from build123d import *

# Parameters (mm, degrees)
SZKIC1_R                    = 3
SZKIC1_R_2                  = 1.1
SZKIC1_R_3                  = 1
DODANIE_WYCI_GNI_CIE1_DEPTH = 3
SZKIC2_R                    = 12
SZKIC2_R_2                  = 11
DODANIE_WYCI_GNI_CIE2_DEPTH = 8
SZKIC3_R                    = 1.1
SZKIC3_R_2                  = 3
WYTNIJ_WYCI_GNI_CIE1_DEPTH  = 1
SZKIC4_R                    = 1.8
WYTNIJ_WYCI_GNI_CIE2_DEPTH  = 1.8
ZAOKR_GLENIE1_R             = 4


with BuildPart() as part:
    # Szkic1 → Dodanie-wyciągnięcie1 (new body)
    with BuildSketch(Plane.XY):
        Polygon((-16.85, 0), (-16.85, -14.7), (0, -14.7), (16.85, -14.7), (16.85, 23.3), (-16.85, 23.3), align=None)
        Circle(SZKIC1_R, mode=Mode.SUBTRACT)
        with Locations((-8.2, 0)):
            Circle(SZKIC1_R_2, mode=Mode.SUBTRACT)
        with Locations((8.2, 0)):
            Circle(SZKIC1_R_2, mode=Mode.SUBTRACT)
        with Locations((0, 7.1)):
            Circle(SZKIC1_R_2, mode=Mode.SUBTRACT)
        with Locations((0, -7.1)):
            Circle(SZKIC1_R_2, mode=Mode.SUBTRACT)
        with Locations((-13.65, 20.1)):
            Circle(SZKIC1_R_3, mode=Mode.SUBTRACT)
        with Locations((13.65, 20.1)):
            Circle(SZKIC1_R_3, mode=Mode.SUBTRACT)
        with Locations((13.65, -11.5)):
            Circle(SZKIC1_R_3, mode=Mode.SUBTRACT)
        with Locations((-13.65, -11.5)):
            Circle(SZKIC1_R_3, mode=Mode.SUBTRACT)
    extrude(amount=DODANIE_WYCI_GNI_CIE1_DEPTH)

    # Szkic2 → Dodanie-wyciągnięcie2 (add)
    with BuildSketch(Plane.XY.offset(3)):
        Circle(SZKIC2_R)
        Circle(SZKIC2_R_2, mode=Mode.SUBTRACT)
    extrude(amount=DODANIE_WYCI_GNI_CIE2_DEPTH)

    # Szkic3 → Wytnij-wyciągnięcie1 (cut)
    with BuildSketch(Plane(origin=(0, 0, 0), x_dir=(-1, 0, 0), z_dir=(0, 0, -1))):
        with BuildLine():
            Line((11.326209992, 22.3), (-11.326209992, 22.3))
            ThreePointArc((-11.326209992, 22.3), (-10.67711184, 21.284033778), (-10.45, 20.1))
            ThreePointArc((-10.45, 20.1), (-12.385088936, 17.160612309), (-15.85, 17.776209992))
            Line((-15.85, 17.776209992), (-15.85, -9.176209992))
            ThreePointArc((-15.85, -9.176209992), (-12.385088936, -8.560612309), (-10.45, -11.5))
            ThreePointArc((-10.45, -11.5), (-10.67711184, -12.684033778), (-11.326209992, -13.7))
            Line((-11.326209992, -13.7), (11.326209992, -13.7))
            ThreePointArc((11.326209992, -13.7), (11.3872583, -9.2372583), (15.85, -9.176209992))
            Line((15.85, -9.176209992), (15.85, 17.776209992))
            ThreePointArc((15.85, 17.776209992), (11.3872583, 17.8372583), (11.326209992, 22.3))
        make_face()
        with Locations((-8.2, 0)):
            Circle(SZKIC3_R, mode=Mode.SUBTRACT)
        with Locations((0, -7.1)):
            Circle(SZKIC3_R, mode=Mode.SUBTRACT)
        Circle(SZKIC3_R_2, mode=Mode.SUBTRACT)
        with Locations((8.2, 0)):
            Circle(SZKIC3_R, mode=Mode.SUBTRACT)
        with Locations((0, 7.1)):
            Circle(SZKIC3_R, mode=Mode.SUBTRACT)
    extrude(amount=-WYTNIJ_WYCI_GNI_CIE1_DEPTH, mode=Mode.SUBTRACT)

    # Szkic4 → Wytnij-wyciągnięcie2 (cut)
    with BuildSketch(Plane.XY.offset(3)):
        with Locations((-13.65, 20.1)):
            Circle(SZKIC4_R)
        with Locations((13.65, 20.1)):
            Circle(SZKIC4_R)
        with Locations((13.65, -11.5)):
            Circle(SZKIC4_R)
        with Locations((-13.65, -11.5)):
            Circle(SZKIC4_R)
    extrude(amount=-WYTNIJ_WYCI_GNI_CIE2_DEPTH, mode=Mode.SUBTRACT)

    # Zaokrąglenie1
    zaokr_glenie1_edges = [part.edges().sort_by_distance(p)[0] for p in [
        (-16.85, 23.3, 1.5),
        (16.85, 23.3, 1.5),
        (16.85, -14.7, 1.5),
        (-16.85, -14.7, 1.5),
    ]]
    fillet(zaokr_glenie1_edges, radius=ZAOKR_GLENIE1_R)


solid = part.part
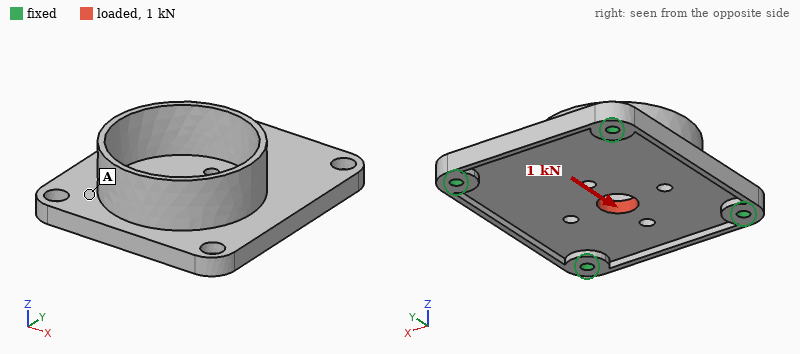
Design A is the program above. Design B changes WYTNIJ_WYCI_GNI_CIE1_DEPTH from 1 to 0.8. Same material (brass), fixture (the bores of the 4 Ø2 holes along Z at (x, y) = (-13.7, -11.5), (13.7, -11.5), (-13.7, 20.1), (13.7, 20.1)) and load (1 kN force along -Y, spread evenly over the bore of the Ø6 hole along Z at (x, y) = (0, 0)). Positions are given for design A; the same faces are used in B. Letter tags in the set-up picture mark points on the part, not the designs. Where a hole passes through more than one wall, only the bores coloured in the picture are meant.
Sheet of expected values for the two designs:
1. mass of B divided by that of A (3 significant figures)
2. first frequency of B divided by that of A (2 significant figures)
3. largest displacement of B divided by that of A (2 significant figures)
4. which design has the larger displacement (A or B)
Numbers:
1.06
1.0
0.90
A
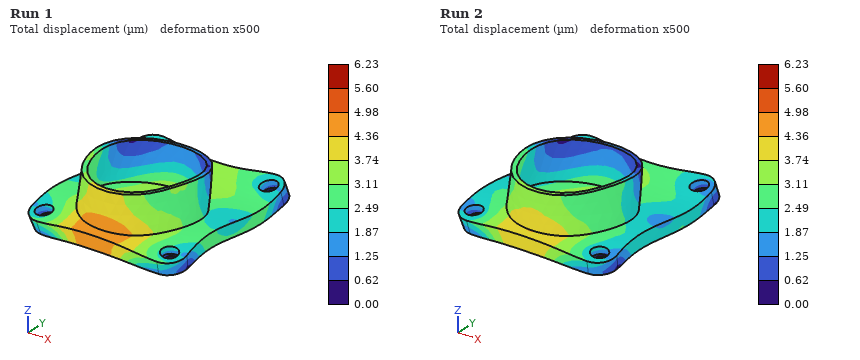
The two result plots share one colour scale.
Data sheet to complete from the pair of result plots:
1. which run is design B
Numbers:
Run 2
